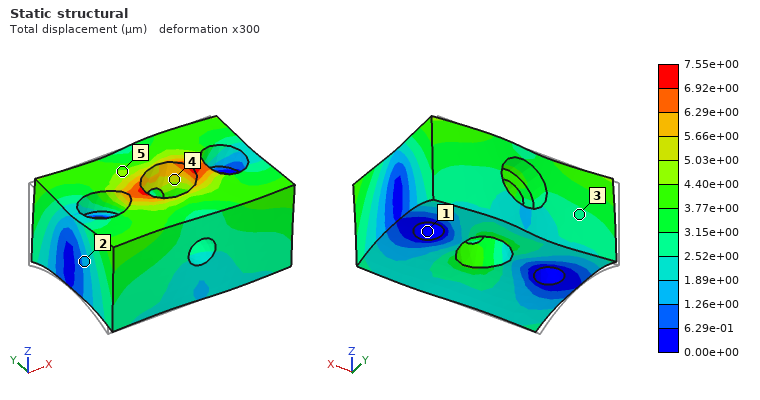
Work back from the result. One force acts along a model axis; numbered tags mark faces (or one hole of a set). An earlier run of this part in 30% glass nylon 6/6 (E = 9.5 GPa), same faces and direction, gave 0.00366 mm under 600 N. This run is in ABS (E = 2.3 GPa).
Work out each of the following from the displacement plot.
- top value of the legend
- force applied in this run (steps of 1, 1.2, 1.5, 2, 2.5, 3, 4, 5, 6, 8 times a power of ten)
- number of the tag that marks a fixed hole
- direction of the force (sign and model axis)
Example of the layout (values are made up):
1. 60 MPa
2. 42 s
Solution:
1. 7.55e+00 µm
2. 300 N
3. 1
4. +X
